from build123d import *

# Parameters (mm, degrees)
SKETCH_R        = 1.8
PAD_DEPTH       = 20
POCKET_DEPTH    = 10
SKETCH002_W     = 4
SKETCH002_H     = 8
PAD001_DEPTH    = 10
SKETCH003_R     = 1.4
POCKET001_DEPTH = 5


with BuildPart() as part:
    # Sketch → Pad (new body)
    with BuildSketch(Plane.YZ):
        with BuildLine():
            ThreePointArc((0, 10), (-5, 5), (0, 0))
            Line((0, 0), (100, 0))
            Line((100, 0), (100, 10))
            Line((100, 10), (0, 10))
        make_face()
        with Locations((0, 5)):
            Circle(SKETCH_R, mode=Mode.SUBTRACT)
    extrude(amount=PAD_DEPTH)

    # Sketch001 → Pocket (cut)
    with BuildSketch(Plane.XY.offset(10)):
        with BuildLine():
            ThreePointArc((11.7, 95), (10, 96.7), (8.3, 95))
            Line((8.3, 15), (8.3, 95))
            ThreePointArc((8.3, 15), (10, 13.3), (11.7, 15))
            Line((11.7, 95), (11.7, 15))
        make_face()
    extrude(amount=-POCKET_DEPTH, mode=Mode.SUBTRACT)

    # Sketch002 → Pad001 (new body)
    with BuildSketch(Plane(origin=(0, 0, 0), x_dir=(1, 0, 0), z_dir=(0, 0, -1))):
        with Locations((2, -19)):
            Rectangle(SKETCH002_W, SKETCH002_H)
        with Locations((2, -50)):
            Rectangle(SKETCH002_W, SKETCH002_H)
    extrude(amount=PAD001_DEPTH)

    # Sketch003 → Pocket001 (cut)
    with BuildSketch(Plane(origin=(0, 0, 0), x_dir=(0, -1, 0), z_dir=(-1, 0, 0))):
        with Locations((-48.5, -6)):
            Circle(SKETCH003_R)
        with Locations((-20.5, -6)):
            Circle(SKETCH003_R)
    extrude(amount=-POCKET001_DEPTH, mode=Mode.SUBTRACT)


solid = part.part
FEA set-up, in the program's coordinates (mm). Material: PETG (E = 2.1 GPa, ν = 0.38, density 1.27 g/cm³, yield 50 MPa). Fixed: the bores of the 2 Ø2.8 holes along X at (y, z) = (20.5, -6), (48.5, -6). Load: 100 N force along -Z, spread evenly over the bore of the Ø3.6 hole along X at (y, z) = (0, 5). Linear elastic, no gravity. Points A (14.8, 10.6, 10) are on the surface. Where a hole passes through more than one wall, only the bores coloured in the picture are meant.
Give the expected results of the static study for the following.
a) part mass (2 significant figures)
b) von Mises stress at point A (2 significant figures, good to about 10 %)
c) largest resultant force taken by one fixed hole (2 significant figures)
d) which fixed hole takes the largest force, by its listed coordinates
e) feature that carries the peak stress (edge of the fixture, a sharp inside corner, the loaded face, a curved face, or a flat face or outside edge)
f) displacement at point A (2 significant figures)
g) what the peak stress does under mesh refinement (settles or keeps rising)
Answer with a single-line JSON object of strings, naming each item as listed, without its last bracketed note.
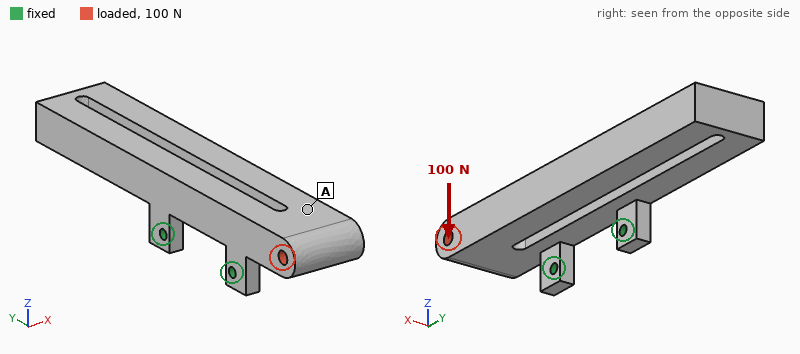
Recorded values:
{"part mass": "23 g", "von Mises stress at point A": "2.5 MPa", "largest resultant force taken by one fixed hole": "160 N", "which fixed hole takes the largest force, by its listed coordinates": "(20.5, -6)", "feature that carries the peak stress": "edge of the fixture", "displacement at point A": "0.84 mm", "what the peak stress does under mesh refinement": "keeps rising"}
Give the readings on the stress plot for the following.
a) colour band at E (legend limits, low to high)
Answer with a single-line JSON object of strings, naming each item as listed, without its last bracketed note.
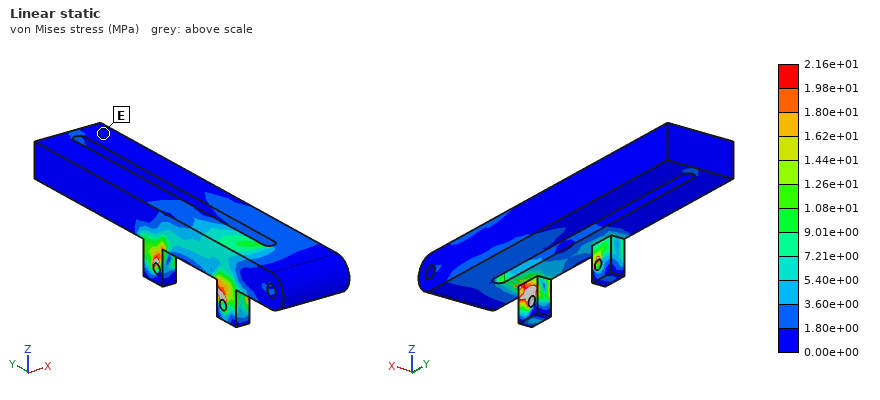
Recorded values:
{"colour band at E": "0.00e+00 to 1.80e+00 MPa"}
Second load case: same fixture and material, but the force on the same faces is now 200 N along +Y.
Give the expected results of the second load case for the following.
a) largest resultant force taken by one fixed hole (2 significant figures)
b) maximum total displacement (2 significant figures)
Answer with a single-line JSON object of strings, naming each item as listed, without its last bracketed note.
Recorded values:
{"largest resultant force taken by one fixed hole": "130 N", "maximum total displacement": "0.74 mm"}
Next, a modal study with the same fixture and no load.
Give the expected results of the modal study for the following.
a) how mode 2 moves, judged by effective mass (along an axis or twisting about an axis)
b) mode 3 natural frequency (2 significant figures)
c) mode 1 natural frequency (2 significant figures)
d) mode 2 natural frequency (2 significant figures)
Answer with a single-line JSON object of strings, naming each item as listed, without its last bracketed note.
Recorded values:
{"how mode 2 moves, judged by effective mass": "along Z", "mode 3 natural frequency": "570 Hz", "mode 1 natural frequency": "300 Hz", "mode 2 natural frequency": "370 Hz"}
